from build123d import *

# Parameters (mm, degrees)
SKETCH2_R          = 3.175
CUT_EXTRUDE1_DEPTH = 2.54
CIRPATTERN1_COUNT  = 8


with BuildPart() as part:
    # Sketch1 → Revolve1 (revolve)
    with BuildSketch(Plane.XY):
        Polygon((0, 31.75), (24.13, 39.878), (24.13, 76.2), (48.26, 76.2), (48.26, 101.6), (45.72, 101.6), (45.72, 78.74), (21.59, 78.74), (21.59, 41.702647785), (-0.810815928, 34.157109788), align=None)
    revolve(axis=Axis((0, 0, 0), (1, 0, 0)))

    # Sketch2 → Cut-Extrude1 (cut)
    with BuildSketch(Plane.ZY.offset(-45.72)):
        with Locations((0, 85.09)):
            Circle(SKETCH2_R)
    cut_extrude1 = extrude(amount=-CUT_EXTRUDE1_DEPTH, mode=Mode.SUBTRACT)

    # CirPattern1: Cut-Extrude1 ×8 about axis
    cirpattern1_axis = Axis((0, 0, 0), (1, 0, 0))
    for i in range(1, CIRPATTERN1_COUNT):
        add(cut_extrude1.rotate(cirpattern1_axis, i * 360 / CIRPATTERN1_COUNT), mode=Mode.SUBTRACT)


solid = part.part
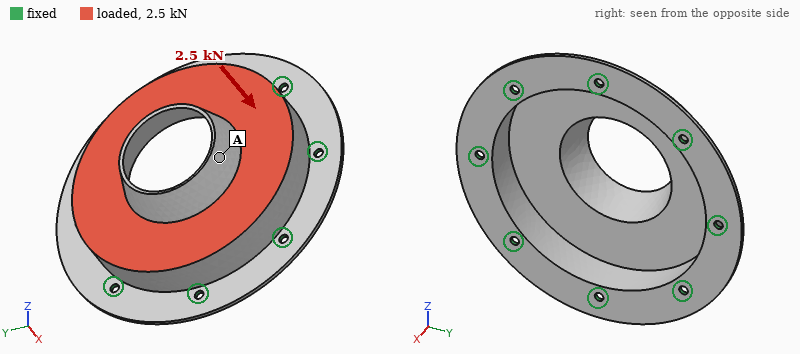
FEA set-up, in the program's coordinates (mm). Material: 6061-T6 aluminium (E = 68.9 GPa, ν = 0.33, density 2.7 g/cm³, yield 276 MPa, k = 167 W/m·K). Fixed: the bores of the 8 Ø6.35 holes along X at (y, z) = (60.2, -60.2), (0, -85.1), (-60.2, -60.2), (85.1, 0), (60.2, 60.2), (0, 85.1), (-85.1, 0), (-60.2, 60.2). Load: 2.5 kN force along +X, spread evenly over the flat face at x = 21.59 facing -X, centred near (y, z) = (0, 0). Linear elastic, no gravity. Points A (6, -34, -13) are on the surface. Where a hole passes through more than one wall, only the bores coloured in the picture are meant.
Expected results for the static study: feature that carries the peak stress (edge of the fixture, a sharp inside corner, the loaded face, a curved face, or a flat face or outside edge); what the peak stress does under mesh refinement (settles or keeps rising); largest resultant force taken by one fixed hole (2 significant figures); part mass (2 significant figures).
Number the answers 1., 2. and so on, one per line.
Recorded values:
1. edge of the fixture
2. keeps rising
3. 330 N
4. 300 g
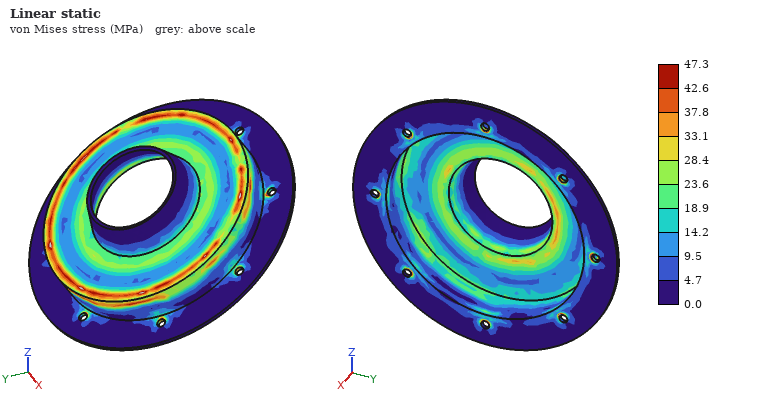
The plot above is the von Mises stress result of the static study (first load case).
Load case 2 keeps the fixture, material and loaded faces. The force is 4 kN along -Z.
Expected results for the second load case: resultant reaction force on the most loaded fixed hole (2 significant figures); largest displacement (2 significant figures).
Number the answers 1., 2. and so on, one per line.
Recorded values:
1. 790 N
2. 27 µm
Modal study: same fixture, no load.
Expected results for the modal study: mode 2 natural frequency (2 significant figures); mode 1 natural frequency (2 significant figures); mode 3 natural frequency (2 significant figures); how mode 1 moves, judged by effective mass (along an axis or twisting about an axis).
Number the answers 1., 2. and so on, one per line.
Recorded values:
1. 2200 Hz
2. 1600 Hz
3. 2200 Hz
4. along X
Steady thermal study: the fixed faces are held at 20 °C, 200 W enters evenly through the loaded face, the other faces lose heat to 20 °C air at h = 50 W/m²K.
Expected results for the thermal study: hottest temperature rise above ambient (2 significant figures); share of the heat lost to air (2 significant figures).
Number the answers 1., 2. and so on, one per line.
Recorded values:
1. 38 K
2. 38 %
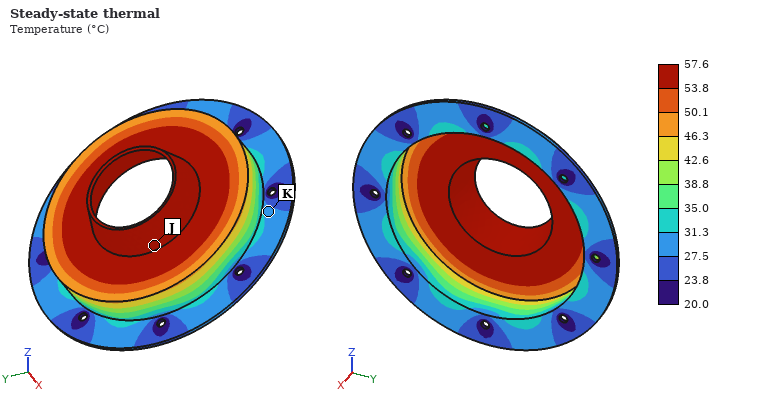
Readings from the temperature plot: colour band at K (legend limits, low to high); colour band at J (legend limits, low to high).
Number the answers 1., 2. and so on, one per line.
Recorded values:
1. 27.5 to 31.3 °C
2. 53.8 to 57.6 °C
